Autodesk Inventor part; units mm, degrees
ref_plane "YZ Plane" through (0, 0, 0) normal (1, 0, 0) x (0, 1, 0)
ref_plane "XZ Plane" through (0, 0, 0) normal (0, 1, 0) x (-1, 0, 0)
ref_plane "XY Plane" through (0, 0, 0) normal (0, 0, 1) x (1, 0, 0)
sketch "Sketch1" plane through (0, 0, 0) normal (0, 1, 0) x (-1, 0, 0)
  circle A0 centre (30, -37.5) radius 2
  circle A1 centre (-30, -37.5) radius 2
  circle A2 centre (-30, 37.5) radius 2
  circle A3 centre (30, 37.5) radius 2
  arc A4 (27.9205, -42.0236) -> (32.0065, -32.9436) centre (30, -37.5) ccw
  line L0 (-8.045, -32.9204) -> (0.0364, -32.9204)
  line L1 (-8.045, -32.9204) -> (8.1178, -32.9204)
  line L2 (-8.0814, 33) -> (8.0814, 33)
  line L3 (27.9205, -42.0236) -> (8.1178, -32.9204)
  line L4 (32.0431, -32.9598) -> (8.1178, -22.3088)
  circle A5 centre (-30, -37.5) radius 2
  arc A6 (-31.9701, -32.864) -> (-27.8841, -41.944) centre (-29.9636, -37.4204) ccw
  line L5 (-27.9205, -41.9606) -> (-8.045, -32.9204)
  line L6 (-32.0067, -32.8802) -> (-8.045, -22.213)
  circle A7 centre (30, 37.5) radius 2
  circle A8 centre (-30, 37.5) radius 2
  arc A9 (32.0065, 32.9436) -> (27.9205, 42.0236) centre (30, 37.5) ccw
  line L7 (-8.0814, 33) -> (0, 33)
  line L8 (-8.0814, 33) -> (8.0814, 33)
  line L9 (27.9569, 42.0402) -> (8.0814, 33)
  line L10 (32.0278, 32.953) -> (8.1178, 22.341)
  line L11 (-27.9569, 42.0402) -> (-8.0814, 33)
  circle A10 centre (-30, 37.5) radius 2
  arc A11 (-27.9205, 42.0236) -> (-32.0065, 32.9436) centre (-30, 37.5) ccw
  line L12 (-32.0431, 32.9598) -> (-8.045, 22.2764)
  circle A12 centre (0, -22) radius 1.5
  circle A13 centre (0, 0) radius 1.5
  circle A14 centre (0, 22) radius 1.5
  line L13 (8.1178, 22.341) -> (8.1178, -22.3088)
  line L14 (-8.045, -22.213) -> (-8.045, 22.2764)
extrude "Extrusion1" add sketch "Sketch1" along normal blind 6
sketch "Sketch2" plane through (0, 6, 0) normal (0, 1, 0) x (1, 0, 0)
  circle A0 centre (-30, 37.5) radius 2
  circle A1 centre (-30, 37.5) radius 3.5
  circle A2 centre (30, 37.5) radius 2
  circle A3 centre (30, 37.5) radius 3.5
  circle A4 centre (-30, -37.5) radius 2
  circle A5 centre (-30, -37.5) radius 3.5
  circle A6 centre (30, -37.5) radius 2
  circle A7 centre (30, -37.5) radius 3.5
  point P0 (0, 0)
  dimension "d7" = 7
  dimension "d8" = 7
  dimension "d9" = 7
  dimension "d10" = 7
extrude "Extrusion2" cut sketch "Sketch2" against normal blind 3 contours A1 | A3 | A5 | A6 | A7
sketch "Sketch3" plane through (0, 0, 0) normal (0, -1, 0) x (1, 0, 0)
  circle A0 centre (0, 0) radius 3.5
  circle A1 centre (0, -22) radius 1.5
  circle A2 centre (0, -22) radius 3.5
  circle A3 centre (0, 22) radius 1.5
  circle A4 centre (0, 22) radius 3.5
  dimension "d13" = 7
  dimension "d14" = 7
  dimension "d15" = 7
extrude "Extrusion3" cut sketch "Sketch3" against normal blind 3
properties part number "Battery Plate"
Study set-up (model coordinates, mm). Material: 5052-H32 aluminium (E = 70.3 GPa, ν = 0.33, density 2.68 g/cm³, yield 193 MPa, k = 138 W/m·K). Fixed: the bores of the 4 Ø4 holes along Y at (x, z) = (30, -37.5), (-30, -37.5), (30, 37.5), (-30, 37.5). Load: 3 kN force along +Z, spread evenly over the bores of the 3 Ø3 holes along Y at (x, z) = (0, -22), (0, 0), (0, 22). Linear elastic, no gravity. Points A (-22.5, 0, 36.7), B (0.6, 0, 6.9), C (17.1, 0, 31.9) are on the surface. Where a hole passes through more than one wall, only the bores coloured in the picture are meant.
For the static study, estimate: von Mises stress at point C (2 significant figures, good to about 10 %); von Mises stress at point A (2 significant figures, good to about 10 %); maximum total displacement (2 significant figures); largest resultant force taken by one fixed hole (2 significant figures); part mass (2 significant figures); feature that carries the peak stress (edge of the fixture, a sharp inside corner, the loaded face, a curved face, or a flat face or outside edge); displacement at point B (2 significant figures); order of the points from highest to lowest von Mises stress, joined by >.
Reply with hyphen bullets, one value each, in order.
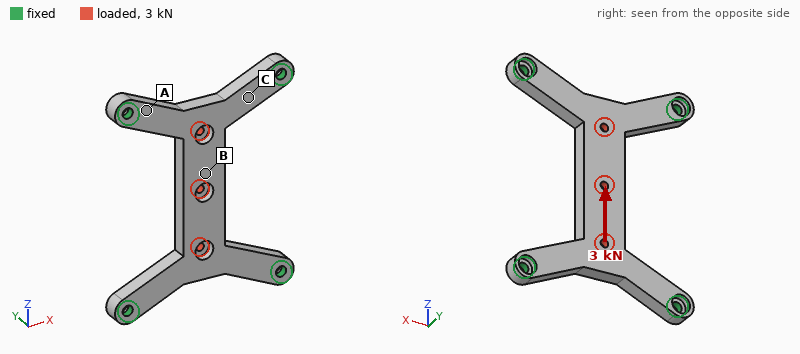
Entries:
- 32 MPa
- 42 MPa
- 34 µm
- 1.3 kN
- 32 g
- edge of the fixture
- 32 µm
- A > C > B
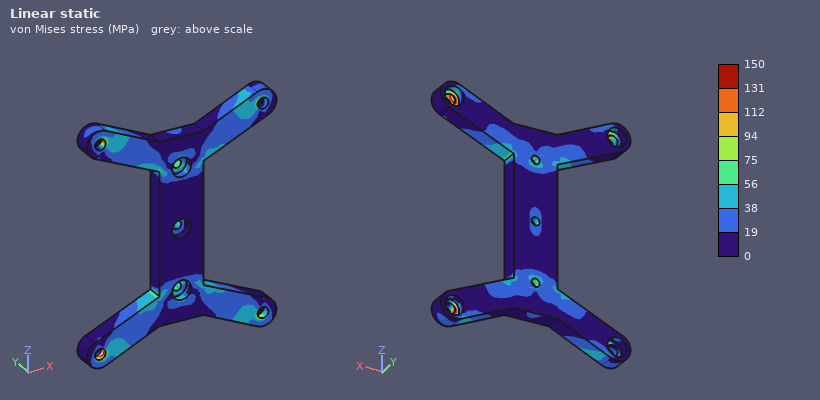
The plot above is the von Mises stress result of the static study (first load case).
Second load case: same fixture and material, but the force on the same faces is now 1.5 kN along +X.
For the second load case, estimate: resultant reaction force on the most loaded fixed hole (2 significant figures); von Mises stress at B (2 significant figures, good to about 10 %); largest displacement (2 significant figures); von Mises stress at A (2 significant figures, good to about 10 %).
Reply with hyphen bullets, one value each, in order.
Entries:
- 440 N
- 3.1 MPa
- 14 µm
- 12 MPa
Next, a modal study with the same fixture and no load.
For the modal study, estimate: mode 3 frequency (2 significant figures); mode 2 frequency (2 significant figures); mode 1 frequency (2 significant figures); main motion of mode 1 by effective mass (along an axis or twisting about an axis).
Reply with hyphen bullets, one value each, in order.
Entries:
- 10 kHz
- 6200 Hz
- 3200 Hz
- along Y
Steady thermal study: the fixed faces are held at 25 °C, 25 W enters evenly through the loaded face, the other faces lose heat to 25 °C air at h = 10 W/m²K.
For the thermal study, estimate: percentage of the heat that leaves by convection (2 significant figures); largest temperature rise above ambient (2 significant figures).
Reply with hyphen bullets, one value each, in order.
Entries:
- 4.4 %
- 35 K
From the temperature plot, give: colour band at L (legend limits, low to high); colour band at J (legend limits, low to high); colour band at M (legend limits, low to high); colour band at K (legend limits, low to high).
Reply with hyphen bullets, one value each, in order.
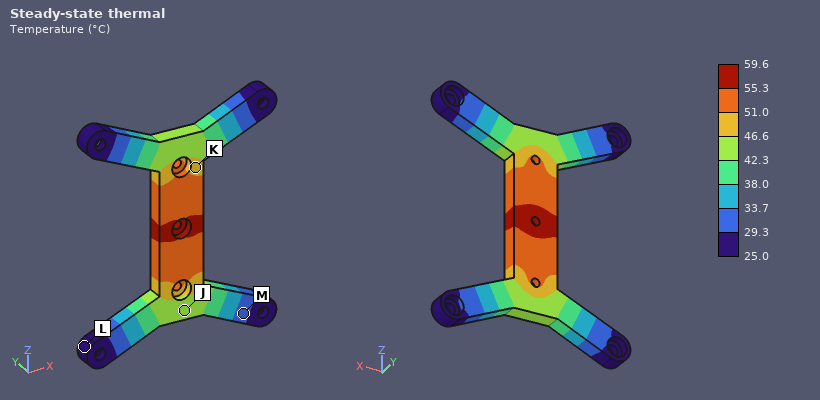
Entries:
- 25.0 to 29.3 °C
- 42.3 to 46.6 °C
- 29.3 to 33.7 °C
- 46.6 to 51.0 °C
